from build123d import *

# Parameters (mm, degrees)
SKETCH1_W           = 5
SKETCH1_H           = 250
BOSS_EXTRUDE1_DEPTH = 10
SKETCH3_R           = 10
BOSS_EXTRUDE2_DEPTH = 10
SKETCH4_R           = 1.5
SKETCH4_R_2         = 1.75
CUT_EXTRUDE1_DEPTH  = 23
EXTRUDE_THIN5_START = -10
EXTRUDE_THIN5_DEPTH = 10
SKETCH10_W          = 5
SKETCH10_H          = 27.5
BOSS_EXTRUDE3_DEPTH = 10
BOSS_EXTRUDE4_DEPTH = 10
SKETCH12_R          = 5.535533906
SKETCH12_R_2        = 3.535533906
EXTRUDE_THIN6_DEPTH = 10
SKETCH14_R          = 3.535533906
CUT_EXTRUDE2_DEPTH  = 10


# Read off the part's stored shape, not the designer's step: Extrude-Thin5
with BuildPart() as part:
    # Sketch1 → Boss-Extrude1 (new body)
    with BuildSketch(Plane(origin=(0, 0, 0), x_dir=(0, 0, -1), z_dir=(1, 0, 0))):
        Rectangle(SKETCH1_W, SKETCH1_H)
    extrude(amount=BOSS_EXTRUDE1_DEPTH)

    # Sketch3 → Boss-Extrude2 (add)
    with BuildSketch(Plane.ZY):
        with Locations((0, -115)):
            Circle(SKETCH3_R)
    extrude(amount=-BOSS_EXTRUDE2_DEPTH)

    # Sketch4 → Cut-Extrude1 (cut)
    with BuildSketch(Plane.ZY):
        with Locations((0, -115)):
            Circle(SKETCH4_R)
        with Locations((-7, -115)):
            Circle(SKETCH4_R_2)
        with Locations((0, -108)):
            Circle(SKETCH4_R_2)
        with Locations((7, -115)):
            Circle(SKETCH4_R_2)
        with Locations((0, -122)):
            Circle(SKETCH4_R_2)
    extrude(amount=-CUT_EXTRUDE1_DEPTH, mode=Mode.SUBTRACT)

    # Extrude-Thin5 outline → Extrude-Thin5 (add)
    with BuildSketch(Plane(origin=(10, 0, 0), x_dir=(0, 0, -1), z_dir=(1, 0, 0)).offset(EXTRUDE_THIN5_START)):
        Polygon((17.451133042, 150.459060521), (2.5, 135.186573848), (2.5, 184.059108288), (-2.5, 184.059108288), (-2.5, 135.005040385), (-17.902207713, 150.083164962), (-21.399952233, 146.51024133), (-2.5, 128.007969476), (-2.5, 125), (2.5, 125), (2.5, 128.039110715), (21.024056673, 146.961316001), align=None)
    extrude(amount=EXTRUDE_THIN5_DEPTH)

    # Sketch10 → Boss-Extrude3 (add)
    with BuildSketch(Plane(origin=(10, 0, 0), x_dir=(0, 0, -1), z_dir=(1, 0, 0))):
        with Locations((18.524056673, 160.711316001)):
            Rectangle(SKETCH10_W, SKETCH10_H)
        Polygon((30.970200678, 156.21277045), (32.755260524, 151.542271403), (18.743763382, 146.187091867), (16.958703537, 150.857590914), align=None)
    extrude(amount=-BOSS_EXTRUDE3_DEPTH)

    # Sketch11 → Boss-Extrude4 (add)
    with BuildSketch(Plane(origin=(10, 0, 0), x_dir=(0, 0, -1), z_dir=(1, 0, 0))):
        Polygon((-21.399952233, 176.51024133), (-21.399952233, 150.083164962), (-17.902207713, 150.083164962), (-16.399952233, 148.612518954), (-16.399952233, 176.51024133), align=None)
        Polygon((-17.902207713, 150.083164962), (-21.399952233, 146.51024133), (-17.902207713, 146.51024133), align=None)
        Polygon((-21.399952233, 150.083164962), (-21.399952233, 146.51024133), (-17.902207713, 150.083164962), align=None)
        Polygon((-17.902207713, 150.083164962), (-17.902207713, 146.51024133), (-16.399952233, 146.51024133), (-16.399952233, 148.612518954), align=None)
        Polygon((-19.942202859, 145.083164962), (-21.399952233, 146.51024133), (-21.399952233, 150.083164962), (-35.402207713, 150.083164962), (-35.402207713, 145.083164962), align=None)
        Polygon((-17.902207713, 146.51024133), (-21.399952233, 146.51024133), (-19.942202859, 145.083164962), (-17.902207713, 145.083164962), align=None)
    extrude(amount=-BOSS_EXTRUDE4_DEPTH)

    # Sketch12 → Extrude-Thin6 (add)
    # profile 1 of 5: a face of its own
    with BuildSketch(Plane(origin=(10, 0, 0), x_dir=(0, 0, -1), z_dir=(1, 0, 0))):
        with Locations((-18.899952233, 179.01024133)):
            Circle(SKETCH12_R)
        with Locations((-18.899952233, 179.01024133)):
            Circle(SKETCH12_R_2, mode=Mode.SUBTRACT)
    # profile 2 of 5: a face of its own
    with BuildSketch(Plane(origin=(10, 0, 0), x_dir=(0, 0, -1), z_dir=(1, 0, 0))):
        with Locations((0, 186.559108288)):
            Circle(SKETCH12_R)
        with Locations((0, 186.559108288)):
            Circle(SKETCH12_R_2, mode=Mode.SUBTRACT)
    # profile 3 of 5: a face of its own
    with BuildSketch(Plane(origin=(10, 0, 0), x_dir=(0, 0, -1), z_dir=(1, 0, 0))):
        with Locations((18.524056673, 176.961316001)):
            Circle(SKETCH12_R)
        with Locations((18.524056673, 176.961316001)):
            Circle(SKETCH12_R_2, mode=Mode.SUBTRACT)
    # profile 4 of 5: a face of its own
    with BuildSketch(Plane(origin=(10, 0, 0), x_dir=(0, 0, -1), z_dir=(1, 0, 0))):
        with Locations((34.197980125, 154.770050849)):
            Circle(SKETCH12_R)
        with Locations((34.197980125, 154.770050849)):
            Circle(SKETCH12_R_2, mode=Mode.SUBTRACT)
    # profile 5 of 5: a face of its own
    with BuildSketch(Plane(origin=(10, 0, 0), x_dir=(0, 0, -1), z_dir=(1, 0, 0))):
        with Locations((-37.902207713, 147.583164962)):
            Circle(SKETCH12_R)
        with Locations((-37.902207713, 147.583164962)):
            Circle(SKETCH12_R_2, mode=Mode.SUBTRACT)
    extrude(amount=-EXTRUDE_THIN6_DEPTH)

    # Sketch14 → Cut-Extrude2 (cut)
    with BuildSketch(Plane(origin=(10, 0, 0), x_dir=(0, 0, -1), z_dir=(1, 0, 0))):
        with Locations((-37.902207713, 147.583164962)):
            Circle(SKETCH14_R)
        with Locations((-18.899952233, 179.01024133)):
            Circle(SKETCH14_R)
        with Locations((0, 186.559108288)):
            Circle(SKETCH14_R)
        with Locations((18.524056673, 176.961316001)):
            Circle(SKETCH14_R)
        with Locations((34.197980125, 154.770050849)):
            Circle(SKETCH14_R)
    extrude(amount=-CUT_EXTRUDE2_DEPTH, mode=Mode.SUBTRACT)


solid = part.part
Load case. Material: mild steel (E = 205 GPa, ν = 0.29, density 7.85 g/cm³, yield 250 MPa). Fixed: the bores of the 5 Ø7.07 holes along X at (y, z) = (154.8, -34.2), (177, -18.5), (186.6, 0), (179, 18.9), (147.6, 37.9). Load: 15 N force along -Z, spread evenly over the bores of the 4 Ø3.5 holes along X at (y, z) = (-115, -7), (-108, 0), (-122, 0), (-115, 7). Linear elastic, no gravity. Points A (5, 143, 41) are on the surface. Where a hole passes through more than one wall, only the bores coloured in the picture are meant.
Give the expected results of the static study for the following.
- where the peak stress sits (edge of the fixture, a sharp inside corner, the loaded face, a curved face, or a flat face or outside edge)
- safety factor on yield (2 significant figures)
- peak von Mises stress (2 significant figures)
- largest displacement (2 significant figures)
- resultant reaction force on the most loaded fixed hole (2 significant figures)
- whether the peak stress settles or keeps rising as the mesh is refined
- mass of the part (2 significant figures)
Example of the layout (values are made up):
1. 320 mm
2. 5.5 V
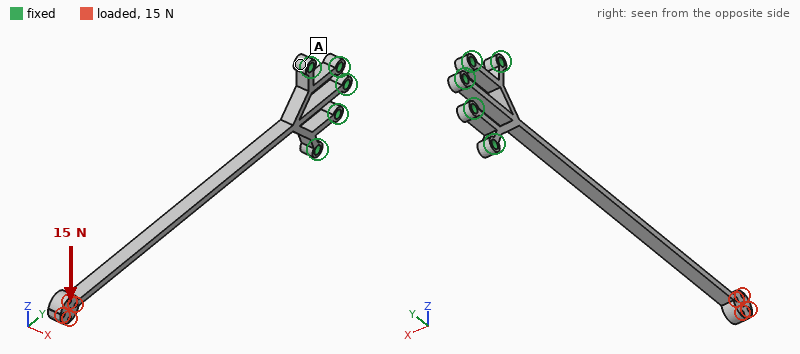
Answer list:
1. a flat face or outside edge
2. 3.0
3. 84 MPa
4. 3.7 mm
5. 130 N
6. settles
7. 200 g
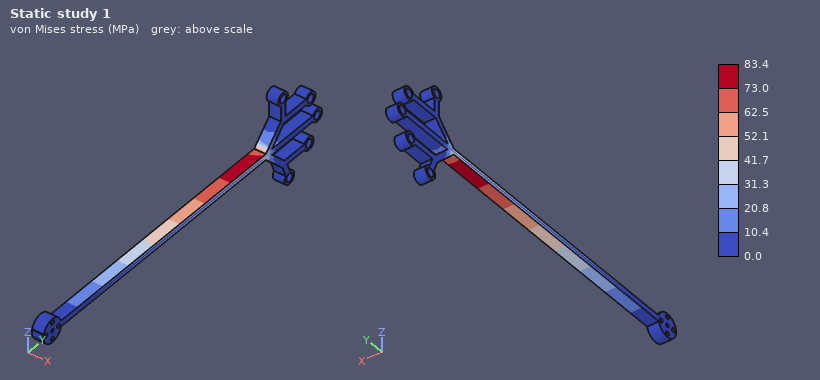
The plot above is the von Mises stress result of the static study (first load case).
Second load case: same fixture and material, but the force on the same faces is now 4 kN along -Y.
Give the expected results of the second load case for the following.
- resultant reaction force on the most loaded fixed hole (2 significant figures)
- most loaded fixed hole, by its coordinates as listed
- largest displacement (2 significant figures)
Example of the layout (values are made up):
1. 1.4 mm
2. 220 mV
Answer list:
1. 1.7 kN
2. (186.6, 0)
3. 0.10 mm
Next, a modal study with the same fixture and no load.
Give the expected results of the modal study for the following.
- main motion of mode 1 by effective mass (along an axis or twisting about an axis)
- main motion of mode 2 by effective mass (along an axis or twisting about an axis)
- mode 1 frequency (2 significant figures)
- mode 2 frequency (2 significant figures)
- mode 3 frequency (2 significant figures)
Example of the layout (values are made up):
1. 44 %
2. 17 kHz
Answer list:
1. along Z
2. along X
3. 52 Hz
4. 94 Hz
5. 350 Hz
